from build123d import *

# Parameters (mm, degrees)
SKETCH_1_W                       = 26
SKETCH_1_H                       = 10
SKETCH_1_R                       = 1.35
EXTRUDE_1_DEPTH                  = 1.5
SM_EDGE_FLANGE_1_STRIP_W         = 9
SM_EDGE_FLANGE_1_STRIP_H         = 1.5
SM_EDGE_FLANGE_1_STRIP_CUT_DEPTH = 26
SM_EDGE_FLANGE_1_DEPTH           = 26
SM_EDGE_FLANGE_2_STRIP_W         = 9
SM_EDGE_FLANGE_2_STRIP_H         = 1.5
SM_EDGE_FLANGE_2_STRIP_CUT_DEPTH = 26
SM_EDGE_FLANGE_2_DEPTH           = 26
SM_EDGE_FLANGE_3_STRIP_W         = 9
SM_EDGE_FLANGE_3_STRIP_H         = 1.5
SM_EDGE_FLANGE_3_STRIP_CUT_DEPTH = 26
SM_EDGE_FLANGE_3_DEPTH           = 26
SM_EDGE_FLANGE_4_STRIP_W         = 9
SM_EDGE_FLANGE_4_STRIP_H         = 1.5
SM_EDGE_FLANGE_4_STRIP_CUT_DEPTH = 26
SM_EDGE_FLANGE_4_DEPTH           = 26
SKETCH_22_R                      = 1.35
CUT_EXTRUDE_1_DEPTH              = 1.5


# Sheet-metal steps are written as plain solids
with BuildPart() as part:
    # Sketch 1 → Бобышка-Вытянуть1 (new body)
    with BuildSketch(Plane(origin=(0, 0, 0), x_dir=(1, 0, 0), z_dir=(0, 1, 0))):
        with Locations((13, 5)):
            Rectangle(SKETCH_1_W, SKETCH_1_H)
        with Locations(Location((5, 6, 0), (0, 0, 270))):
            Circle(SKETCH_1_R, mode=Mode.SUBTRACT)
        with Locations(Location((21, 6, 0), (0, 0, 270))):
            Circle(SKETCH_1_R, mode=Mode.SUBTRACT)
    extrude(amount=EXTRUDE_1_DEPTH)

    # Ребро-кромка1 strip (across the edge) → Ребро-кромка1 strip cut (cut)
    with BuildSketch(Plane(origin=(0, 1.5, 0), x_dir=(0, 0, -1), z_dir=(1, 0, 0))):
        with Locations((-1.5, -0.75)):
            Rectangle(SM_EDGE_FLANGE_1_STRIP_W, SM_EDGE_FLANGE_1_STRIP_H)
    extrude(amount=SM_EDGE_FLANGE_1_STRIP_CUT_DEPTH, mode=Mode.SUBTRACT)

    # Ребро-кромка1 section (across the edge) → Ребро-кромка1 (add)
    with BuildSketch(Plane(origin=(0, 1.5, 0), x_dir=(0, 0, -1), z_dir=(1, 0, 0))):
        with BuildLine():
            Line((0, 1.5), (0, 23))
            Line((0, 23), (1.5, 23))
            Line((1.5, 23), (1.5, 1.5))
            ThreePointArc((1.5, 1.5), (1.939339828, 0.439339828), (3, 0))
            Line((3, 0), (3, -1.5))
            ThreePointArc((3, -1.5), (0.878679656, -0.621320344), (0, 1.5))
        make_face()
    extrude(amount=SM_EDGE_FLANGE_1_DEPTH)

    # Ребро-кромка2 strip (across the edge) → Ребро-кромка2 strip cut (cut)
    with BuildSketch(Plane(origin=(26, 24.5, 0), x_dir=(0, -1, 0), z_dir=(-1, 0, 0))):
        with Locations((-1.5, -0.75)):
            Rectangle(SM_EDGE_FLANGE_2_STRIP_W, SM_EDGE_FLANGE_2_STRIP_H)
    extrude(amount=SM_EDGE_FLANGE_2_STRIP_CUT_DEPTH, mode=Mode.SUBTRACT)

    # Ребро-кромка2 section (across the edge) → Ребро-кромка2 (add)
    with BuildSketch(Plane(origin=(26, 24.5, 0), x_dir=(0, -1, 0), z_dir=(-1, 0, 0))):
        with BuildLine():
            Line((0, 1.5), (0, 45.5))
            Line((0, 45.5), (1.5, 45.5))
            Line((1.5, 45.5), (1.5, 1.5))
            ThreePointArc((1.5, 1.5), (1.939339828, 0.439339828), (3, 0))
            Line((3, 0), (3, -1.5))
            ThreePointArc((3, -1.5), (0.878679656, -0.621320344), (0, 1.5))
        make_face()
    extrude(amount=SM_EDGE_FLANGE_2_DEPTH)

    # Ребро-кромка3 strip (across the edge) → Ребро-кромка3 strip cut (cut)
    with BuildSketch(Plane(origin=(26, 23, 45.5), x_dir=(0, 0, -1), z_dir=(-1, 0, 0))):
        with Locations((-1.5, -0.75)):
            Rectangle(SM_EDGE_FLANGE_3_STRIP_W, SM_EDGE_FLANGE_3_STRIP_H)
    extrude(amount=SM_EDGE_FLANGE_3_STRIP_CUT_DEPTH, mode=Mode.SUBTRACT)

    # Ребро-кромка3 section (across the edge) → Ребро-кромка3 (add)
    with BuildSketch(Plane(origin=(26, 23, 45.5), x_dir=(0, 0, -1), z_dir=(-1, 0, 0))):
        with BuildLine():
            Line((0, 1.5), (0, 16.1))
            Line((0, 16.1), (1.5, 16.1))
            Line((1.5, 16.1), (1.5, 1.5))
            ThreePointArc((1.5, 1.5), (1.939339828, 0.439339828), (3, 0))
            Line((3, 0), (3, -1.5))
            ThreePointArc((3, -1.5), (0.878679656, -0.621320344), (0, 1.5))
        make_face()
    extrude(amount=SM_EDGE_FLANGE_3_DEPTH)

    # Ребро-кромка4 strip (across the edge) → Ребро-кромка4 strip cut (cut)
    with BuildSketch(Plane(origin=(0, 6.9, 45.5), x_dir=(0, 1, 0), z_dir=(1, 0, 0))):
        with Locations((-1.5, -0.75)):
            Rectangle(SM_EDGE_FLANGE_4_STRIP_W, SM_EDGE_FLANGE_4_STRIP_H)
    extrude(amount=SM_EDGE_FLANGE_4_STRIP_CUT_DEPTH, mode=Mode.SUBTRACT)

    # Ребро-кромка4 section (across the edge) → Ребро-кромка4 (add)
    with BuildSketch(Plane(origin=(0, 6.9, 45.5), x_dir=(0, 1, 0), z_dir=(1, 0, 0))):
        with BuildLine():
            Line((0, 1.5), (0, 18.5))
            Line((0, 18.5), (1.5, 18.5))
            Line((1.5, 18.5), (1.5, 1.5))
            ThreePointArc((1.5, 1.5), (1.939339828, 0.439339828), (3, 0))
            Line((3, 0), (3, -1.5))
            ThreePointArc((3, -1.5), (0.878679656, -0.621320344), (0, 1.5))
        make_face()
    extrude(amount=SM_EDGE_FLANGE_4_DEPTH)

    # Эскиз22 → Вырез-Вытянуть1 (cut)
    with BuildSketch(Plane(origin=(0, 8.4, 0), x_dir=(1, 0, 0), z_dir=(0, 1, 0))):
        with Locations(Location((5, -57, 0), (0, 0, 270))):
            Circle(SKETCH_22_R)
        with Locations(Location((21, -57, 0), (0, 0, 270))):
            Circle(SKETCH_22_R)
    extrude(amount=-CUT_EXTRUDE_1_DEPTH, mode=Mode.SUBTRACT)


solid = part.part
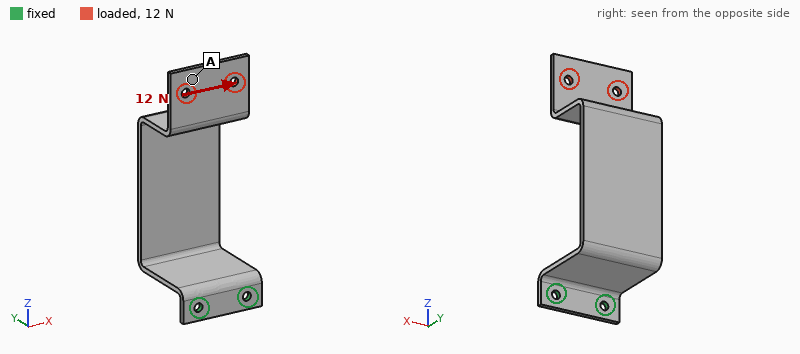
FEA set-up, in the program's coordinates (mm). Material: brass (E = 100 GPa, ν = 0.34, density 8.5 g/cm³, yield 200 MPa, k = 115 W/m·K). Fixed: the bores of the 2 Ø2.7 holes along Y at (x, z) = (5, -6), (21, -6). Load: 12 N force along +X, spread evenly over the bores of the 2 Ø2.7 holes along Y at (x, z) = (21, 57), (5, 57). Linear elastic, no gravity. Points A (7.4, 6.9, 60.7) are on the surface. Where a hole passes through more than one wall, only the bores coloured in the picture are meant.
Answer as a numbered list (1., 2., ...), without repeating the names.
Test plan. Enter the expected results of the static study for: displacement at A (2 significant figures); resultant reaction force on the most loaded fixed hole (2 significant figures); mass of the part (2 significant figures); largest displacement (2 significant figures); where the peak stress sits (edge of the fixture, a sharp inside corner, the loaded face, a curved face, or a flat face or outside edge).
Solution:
1. 0.84 mm
2. 42 N
3. 36 g
4. 0.89 mm
5. a curved face
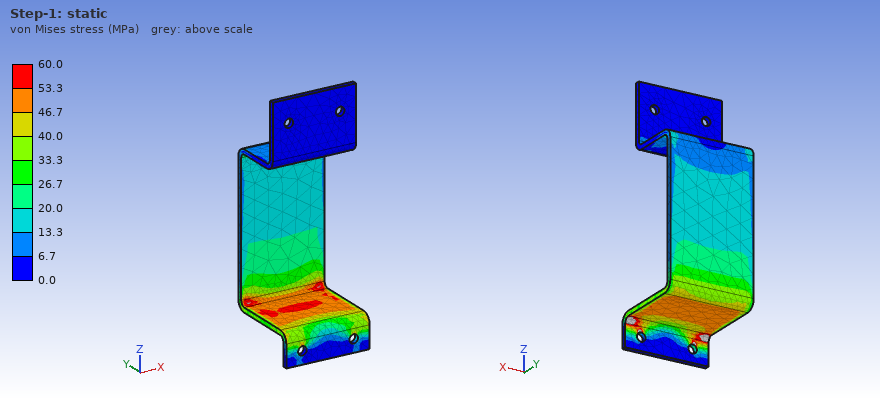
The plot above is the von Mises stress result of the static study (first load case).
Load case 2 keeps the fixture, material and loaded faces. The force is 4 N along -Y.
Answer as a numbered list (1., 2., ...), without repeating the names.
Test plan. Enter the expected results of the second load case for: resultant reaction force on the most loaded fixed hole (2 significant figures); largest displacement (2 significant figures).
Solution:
1. 3.1 N
2. 0.93 mm
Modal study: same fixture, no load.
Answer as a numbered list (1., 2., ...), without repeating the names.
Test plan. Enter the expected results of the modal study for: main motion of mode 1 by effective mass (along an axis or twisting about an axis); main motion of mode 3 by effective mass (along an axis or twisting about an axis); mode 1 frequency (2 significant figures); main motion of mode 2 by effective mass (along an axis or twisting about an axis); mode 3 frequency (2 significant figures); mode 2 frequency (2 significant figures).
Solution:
1. along Y
2. along Z
3. 110 Hz
4. along X
5. 380 Hz
6. 190 Hz
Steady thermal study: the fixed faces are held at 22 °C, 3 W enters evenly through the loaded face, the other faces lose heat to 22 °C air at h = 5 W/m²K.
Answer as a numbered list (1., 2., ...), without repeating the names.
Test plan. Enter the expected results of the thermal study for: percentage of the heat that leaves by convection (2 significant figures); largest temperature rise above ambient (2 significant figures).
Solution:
1. 27 %
2. 55 K
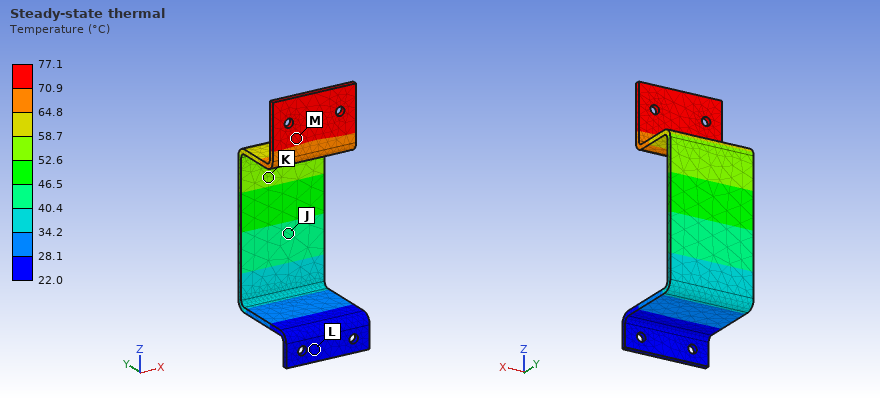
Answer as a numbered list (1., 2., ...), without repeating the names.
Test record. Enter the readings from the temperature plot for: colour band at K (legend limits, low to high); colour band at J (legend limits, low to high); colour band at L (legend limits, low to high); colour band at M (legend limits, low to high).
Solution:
1. 52.6 to 58.7 °C
2. 40.4 to 46.5 °C
3. 22.0 to 28.1 °C
4. 70.9 to 77.1 °C
